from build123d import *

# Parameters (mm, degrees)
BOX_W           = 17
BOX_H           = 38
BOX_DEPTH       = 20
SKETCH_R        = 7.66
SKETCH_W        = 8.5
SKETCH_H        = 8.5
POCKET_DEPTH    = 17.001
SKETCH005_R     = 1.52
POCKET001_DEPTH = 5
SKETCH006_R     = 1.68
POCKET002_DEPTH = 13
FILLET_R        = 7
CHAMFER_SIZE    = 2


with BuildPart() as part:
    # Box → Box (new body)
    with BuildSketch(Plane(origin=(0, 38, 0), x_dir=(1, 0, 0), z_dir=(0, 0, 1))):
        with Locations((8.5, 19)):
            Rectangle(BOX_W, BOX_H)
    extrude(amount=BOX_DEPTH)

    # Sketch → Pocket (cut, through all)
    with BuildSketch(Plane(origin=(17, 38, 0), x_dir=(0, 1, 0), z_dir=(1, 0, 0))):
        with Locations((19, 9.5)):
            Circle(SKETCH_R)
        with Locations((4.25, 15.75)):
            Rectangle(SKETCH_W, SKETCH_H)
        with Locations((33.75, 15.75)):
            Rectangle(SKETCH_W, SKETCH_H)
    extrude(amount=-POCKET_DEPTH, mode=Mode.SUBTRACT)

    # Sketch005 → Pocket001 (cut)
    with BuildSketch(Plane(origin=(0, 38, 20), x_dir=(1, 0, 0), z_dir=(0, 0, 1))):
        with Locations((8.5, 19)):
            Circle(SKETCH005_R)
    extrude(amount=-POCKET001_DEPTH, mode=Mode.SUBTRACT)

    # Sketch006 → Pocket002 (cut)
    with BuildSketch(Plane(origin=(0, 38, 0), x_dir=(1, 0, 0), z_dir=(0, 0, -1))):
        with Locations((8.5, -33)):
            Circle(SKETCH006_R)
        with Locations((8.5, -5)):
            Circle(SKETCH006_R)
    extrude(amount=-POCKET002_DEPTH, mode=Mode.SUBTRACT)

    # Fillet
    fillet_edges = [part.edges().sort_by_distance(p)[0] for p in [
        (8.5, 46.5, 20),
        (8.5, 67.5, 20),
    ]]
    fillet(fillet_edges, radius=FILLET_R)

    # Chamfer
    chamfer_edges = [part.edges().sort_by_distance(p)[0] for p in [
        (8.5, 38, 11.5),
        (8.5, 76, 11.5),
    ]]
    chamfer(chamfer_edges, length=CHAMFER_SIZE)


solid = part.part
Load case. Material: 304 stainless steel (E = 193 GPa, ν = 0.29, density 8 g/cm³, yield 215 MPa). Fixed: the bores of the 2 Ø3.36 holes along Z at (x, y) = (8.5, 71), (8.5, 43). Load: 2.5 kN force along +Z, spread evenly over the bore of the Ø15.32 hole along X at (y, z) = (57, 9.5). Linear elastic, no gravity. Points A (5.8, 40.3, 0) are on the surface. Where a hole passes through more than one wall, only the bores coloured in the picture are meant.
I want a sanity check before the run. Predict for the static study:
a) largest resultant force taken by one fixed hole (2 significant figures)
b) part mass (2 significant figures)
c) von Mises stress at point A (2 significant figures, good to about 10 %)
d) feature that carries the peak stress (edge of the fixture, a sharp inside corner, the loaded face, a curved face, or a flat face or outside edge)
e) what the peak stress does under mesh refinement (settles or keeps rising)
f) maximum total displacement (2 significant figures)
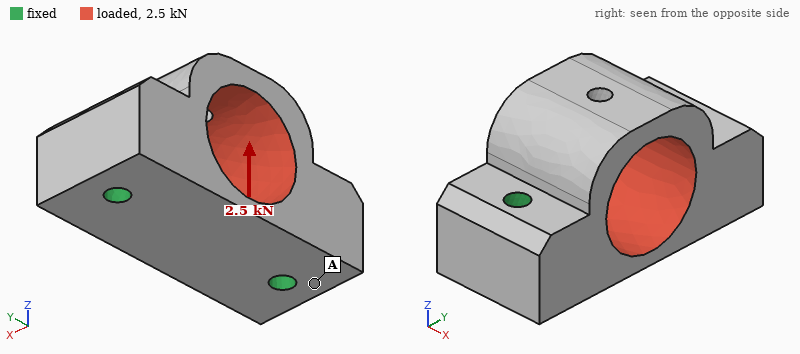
1.3 kN
53 g
8.3 MPa
edge of the fixture
keeps rising
2.3 µm
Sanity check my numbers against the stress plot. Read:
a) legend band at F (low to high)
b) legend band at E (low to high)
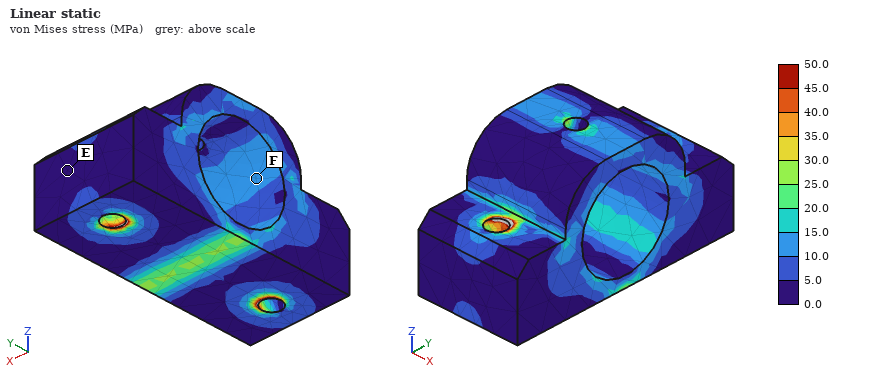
10.0 to 15.0 MPa
0.0 to 5.0 MPa
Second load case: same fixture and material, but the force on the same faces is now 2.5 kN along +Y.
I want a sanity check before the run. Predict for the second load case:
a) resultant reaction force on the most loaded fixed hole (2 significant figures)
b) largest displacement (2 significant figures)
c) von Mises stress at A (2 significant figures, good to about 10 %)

1.3 kN
2.6 µm
3.5 MPa
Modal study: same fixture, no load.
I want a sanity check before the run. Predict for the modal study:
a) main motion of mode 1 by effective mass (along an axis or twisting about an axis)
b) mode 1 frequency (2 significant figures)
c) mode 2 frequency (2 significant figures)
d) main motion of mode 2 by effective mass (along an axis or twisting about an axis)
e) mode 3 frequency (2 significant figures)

along X
24 kHz
30 kHz
along Y
37 kHz
